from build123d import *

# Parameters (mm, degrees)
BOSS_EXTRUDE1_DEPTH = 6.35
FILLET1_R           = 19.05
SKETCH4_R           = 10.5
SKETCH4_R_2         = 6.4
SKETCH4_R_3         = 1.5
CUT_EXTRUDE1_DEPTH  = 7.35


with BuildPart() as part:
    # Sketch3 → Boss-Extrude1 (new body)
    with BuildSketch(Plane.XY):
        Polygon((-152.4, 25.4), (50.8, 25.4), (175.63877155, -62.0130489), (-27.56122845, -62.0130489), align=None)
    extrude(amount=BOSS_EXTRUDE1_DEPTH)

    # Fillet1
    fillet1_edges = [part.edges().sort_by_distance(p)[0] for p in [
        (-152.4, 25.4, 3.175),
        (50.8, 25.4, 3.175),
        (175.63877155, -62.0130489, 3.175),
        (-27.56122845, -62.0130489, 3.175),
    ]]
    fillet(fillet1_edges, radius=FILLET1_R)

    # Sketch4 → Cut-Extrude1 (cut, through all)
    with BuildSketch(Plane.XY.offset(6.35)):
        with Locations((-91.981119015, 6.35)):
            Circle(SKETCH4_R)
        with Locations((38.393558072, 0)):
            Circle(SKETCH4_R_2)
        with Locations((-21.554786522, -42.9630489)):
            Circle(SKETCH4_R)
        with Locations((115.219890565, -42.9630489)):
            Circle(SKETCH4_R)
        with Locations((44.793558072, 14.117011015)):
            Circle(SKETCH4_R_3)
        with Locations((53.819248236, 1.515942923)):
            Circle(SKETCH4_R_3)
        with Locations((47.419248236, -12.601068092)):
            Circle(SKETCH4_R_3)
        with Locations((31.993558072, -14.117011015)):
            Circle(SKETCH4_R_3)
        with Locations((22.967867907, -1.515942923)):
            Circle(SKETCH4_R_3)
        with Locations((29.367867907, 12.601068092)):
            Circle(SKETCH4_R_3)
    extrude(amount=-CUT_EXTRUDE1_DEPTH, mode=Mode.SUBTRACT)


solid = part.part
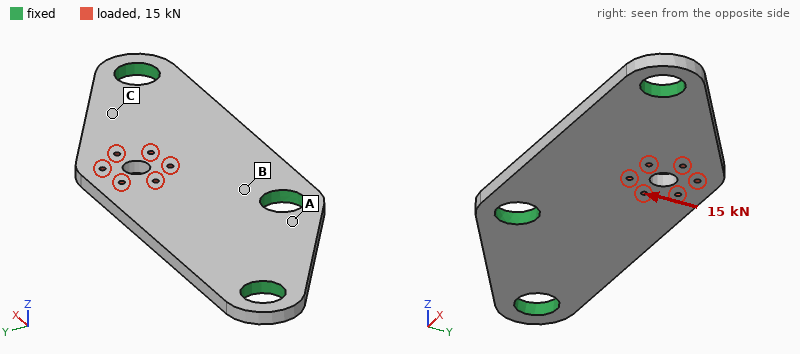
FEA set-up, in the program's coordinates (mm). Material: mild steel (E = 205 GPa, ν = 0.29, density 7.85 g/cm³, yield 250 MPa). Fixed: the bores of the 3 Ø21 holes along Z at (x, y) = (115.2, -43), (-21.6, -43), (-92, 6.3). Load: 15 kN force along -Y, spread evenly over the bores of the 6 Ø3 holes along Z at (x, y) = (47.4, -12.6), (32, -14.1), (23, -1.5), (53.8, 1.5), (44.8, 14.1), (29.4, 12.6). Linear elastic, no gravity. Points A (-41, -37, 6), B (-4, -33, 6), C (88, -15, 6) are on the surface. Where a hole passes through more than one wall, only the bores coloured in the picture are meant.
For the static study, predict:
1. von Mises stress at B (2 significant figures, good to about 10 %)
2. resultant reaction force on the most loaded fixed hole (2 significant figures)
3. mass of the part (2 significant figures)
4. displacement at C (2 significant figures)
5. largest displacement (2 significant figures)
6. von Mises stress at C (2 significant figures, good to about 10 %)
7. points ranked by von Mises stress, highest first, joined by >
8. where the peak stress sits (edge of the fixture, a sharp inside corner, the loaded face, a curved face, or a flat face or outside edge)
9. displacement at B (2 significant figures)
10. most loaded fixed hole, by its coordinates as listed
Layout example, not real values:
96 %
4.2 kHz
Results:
49 MPa
10 kN
760 g
8.6 µm
20 µm
30 MPa
B > C > A
the loaded face
4.4 µm
(-21.6, -43)
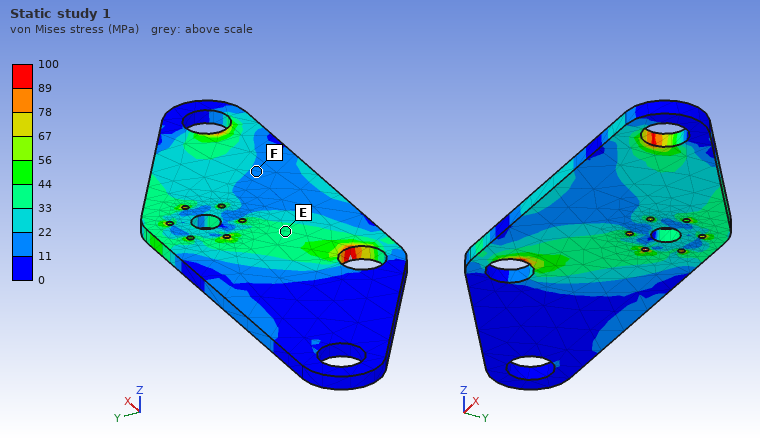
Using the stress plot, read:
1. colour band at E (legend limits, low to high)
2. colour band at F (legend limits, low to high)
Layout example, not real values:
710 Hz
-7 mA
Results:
33 to 44 MPa
11 to 22 MPa
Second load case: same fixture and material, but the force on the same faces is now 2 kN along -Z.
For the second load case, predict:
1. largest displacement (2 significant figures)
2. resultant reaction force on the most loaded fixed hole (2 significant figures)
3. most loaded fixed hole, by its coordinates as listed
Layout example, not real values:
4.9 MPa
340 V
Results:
0.28 mm
1.2 kN
(-21.6, -43)
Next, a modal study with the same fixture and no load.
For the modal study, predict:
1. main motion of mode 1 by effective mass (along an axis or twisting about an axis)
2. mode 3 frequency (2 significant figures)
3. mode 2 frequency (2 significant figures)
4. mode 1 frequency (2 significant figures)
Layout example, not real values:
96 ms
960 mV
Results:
along Z
2900 Hz
2400 Hz
1200 Hz
